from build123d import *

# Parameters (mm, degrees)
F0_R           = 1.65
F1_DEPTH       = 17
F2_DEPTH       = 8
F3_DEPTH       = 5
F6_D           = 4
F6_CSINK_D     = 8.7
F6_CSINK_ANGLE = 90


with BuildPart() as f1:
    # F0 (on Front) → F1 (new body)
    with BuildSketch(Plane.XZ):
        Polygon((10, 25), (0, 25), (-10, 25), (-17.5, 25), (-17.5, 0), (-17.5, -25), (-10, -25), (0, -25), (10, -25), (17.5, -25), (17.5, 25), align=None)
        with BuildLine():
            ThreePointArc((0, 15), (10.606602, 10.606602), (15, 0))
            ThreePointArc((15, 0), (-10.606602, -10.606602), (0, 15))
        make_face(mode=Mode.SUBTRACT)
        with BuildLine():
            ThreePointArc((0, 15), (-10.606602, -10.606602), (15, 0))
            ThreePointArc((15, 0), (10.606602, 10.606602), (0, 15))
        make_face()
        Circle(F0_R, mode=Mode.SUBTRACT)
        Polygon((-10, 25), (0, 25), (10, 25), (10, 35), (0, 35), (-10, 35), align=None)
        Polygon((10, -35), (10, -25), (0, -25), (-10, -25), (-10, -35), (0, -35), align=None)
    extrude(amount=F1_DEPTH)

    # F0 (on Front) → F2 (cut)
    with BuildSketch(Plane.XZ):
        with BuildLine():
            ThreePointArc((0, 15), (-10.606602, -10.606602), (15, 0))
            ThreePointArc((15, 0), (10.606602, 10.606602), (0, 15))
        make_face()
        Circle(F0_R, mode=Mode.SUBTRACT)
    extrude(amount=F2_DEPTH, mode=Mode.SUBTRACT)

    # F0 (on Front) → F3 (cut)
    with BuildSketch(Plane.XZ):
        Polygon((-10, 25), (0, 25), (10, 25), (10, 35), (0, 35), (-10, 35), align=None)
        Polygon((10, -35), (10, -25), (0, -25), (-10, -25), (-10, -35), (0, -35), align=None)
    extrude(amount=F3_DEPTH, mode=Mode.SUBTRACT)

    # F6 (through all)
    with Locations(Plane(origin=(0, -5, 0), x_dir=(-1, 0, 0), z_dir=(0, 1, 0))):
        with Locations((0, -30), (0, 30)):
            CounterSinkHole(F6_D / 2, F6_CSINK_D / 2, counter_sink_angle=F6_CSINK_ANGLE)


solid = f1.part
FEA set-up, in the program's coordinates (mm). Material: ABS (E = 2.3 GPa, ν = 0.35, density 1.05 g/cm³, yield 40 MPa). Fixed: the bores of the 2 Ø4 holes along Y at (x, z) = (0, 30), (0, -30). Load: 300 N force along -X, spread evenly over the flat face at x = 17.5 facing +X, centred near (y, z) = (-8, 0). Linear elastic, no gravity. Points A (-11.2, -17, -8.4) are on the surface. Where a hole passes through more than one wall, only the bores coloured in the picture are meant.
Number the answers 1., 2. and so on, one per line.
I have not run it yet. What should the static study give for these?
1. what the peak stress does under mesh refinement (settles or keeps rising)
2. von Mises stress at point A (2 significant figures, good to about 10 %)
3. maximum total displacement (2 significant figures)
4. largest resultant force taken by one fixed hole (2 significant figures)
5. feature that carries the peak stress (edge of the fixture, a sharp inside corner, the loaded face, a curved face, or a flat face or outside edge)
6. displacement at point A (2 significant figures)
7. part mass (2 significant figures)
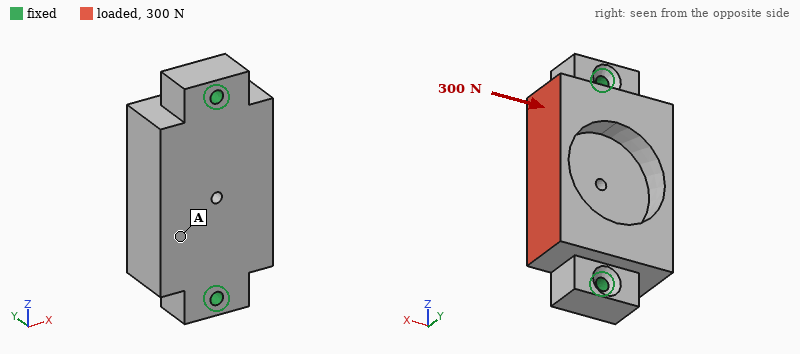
1. keeps rising
2. 0.53 MPa
3. 55 µm
4. 150 N
5. edge of the fixture
6. 13 µm
7. 30 g
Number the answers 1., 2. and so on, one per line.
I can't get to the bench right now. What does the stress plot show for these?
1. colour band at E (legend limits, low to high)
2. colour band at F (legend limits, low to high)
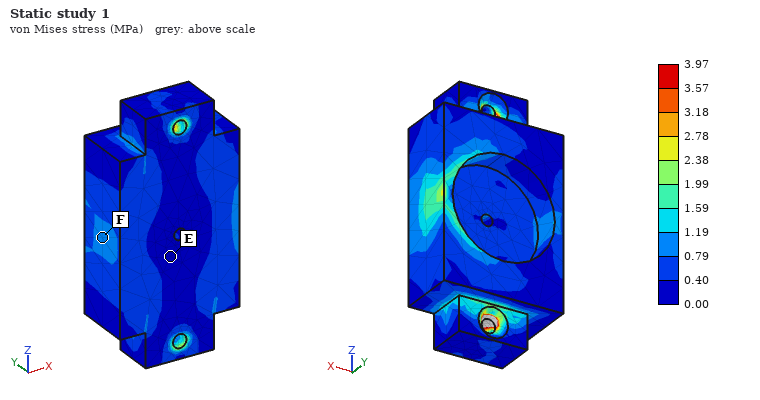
1. 0.00 to 0.40 MPa
2. 0.79 to 1.19 MPa
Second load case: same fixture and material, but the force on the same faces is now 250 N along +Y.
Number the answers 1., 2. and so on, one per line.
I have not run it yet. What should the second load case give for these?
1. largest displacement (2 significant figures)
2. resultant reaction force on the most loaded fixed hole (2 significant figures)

1. 0.17 mm
2. 130 N
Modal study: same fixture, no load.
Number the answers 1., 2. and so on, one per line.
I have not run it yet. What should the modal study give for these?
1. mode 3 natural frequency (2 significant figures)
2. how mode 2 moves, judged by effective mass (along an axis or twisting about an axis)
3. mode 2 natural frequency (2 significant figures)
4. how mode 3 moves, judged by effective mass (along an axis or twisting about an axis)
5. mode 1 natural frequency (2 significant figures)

1. 4600 Hz
2. along Y
3. 2800 Hz
4. along X
5. 2600 Hz
